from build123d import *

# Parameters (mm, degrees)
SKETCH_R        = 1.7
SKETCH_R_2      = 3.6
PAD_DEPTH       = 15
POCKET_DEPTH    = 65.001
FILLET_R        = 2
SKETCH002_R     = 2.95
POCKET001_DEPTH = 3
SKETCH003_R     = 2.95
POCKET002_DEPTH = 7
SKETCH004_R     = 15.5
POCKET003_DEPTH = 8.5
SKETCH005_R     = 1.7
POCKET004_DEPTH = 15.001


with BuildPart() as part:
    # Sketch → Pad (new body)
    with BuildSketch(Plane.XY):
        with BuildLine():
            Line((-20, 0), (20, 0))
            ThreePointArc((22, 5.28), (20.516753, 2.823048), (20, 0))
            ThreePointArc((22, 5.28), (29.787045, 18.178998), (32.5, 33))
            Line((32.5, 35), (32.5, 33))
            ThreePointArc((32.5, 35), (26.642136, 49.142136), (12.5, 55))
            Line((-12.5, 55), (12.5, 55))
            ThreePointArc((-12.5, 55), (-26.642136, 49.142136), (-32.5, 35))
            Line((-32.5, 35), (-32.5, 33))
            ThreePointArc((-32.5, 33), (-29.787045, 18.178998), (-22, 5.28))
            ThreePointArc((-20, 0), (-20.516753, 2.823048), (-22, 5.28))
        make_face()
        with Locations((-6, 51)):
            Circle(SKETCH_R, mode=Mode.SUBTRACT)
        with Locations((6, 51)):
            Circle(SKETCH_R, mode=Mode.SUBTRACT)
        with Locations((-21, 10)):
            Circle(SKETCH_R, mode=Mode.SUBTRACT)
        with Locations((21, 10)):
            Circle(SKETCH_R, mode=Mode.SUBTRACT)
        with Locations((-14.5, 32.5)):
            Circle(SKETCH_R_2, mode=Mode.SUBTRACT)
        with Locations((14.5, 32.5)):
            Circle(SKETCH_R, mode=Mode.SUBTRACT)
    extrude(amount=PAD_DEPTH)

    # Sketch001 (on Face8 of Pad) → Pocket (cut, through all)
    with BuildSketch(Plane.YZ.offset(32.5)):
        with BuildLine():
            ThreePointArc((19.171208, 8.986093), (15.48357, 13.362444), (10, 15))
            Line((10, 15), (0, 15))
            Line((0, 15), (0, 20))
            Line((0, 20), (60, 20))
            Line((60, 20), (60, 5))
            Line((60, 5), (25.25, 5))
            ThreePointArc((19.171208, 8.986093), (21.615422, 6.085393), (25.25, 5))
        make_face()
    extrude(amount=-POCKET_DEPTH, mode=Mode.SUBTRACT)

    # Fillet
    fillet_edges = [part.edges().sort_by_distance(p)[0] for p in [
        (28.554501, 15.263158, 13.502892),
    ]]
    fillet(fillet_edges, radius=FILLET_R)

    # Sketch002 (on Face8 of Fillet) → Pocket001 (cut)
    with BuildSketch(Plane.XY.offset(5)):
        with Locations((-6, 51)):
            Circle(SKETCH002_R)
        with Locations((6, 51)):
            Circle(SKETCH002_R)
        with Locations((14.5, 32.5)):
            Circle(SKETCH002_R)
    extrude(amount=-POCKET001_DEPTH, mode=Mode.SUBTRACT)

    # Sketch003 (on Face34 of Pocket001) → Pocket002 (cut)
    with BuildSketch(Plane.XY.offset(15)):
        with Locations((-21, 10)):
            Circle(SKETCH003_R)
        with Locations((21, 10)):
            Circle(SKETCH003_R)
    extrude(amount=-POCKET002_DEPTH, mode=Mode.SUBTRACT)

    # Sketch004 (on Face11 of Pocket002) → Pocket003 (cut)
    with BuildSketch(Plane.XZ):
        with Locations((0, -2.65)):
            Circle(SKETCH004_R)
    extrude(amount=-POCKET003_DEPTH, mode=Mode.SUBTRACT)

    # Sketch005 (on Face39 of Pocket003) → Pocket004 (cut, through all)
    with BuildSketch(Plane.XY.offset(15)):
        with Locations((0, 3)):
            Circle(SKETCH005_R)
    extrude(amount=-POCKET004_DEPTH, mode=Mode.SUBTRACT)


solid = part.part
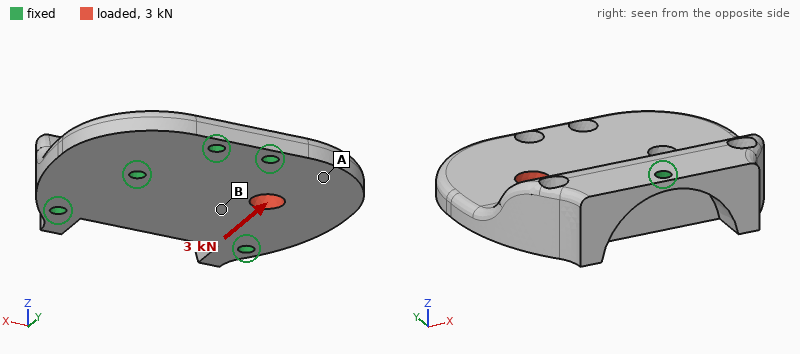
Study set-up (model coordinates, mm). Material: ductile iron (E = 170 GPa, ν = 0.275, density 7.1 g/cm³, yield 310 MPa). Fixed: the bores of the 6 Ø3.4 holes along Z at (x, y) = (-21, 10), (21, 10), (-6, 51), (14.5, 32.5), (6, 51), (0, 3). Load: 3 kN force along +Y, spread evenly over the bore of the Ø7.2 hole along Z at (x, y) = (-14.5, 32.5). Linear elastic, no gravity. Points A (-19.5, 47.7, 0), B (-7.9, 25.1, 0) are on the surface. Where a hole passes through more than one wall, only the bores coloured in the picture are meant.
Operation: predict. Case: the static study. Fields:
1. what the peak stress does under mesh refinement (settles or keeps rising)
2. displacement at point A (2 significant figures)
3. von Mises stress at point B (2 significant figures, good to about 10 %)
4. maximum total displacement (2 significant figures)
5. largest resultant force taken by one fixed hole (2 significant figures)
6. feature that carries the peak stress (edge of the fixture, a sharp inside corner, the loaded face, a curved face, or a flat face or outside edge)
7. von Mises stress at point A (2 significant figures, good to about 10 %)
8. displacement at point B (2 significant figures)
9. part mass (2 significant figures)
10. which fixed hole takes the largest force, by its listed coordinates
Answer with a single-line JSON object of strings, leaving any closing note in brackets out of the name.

{"what the peak stress does under mesh refinement": "keeps rising", "displacement at point A": "2.7 µm", "von Mises stress at point B": "13 MPa", "maximum total displacement": "4.1 µm", "largest resultant force taken by one fixed hole": "1.6 kN", "feature that carries the peak stress": "edge of the fixture", "von Mises stress at point A": "5.5 MPa", "displacement at point B": "2.4 µm", "part mass": "150 g", "which fixed hole takes the largest force, by its listed coordinates": "(-21, 10)"}
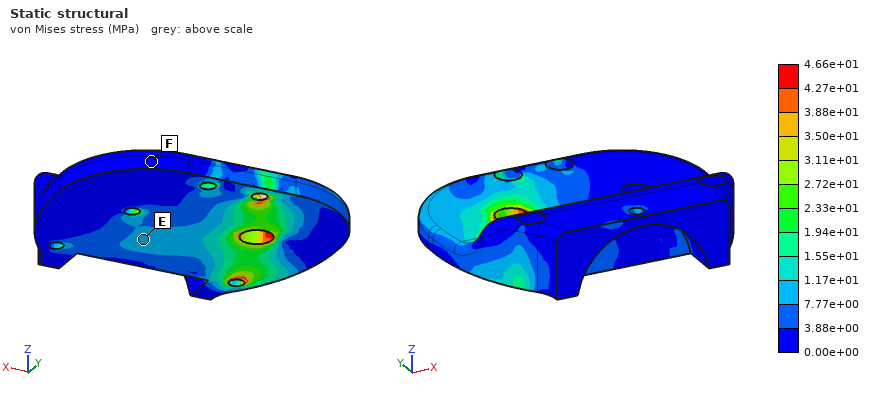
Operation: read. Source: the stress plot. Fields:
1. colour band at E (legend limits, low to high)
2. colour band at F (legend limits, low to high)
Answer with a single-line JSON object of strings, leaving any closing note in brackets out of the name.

{"colour band at E": "7.77e+00 to 1.17e+01 MPa", "colour band at F": "0.00e+00 to 3.88e+00 MPa"}
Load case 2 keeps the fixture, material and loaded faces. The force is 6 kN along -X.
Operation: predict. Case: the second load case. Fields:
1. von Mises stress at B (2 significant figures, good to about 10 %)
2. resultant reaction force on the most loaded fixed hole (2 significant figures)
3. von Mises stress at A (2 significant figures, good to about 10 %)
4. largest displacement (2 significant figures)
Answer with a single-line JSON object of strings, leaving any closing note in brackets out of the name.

{"von Mises stress at B": "35 MPa", "resultant reaction force on the most loaded fixed hole": "1.4 kN", "von Mises stress at A": "23 MPa", "largest displacement": "7.0 µm"}
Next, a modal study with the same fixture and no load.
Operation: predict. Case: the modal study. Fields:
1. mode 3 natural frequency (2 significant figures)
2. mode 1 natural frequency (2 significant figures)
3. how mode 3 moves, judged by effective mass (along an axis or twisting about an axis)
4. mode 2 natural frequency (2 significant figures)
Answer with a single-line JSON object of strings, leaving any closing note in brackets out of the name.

{"mode 3 natural frequency": "16 kHz", "mode 1 natural frequency": "8400 Hz", "how mode 3 moves, judged by effective mass": "along Z", "mode 2 natural frequency": "11 kHz"}
